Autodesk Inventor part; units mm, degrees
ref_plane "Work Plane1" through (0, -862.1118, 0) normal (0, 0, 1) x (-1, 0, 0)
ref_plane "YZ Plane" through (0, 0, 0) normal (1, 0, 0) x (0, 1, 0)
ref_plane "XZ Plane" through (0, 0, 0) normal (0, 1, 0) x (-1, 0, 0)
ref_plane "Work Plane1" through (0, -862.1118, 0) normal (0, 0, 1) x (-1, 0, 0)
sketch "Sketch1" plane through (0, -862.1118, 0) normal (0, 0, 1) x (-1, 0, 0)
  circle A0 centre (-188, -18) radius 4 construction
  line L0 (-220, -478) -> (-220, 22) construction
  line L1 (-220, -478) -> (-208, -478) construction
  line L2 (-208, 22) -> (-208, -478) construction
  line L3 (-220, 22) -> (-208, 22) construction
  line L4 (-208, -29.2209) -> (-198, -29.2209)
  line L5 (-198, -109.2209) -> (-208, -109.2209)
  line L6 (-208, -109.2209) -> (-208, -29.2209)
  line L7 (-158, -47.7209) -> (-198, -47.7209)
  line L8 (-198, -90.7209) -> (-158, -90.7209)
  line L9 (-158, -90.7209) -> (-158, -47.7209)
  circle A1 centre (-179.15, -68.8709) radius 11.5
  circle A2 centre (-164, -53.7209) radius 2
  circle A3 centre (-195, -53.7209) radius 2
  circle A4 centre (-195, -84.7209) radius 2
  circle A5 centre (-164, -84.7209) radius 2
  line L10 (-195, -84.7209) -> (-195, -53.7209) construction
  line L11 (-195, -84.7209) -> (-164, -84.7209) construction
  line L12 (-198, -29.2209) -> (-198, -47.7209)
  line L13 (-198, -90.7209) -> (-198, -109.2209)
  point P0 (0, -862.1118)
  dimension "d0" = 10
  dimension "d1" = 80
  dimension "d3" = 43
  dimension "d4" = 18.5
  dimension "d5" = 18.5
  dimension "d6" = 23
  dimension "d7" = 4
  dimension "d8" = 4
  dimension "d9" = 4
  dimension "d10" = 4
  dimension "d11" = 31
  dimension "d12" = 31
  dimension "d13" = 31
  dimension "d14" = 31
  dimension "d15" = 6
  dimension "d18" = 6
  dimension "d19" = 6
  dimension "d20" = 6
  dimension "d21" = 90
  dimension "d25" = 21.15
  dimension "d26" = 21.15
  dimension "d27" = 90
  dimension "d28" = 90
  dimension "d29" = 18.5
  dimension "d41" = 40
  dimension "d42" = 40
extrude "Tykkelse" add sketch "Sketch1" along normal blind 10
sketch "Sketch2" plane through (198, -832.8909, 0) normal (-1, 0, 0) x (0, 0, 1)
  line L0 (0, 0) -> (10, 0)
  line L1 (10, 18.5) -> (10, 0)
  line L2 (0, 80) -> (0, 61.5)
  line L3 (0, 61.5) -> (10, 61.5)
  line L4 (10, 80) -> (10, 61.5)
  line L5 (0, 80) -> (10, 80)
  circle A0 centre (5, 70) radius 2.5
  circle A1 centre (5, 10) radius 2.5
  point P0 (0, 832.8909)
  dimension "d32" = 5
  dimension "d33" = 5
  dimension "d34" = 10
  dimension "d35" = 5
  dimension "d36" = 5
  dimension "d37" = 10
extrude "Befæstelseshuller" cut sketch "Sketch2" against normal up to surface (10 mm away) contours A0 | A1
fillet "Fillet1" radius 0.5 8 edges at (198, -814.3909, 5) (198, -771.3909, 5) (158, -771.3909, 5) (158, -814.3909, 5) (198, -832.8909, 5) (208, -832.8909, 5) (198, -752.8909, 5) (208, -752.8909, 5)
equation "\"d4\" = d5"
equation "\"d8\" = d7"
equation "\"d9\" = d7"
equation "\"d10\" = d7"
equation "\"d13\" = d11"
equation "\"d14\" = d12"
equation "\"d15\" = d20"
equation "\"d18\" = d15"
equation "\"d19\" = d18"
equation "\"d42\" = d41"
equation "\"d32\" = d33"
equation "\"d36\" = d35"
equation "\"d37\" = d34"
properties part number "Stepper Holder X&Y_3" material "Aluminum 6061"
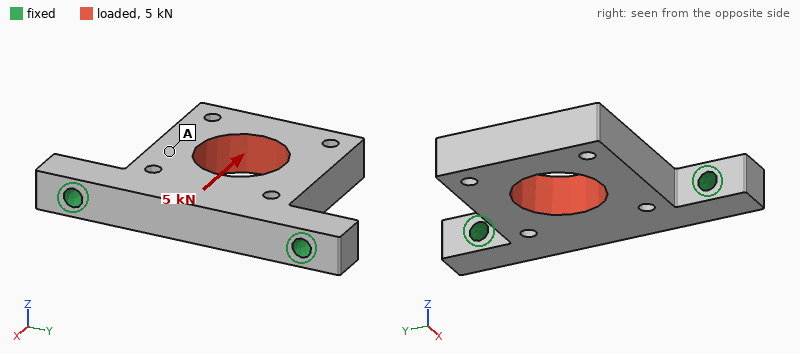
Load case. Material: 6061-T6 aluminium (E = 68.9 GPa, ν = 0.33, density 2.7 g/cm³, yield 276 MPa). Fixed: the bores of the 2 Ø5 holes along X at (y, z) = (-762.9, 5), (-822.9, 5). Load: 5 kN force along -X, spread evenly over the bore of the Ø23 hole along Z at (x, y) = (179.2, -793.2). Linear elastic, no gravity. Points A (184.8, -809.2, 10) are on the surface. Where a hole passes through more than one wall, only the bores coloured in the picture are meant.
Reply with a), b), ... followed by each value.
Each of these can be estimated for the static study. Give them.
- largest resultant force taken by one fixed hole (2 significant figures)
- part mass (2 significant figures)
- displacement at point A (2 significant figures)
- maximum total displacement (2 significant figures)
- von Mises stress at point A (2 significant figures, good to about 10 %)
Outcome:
a) 2.7 kN
b) 54 g
c) 23 µm
d) 29 µm
e) 22 MPa
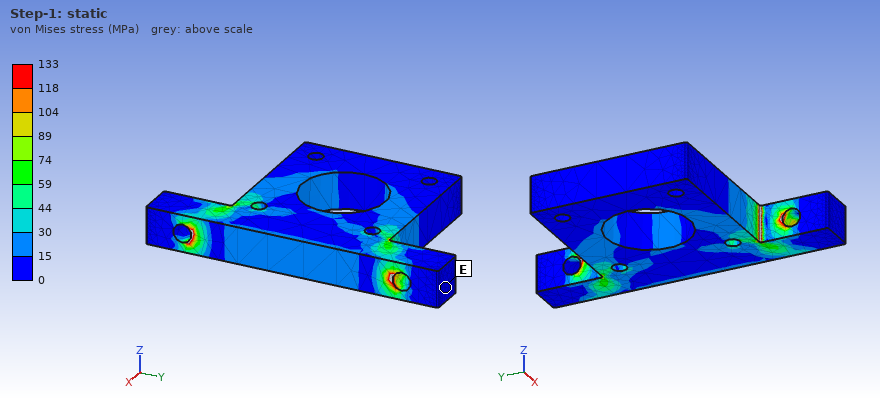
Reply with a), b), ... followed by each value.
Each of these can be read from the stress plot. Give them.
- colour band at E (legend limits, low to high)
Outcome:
a) 0 to 15 MPa
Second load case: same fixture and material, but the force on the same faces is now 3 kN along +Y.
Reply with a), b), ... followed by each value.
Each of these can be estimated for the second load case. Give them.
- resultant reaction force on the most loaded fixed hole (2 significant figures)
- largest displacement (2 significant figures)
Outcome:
a) 2.1 kN
b) 48 µm
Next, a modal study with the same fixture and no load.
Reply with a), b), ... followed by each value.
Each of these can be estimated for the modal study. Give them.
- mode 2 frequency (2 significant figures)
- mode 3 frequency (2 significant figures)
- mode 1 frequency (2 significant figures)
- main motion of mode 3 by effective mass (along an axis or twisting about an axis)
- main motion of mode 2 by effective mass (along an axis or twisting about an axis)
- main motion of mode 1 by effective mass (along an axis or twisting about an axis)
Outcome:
a) 6500 Hz
b) 7300 Hz
c) 2100 Hz
d) along Y
e) twisting about X
f) along Z
